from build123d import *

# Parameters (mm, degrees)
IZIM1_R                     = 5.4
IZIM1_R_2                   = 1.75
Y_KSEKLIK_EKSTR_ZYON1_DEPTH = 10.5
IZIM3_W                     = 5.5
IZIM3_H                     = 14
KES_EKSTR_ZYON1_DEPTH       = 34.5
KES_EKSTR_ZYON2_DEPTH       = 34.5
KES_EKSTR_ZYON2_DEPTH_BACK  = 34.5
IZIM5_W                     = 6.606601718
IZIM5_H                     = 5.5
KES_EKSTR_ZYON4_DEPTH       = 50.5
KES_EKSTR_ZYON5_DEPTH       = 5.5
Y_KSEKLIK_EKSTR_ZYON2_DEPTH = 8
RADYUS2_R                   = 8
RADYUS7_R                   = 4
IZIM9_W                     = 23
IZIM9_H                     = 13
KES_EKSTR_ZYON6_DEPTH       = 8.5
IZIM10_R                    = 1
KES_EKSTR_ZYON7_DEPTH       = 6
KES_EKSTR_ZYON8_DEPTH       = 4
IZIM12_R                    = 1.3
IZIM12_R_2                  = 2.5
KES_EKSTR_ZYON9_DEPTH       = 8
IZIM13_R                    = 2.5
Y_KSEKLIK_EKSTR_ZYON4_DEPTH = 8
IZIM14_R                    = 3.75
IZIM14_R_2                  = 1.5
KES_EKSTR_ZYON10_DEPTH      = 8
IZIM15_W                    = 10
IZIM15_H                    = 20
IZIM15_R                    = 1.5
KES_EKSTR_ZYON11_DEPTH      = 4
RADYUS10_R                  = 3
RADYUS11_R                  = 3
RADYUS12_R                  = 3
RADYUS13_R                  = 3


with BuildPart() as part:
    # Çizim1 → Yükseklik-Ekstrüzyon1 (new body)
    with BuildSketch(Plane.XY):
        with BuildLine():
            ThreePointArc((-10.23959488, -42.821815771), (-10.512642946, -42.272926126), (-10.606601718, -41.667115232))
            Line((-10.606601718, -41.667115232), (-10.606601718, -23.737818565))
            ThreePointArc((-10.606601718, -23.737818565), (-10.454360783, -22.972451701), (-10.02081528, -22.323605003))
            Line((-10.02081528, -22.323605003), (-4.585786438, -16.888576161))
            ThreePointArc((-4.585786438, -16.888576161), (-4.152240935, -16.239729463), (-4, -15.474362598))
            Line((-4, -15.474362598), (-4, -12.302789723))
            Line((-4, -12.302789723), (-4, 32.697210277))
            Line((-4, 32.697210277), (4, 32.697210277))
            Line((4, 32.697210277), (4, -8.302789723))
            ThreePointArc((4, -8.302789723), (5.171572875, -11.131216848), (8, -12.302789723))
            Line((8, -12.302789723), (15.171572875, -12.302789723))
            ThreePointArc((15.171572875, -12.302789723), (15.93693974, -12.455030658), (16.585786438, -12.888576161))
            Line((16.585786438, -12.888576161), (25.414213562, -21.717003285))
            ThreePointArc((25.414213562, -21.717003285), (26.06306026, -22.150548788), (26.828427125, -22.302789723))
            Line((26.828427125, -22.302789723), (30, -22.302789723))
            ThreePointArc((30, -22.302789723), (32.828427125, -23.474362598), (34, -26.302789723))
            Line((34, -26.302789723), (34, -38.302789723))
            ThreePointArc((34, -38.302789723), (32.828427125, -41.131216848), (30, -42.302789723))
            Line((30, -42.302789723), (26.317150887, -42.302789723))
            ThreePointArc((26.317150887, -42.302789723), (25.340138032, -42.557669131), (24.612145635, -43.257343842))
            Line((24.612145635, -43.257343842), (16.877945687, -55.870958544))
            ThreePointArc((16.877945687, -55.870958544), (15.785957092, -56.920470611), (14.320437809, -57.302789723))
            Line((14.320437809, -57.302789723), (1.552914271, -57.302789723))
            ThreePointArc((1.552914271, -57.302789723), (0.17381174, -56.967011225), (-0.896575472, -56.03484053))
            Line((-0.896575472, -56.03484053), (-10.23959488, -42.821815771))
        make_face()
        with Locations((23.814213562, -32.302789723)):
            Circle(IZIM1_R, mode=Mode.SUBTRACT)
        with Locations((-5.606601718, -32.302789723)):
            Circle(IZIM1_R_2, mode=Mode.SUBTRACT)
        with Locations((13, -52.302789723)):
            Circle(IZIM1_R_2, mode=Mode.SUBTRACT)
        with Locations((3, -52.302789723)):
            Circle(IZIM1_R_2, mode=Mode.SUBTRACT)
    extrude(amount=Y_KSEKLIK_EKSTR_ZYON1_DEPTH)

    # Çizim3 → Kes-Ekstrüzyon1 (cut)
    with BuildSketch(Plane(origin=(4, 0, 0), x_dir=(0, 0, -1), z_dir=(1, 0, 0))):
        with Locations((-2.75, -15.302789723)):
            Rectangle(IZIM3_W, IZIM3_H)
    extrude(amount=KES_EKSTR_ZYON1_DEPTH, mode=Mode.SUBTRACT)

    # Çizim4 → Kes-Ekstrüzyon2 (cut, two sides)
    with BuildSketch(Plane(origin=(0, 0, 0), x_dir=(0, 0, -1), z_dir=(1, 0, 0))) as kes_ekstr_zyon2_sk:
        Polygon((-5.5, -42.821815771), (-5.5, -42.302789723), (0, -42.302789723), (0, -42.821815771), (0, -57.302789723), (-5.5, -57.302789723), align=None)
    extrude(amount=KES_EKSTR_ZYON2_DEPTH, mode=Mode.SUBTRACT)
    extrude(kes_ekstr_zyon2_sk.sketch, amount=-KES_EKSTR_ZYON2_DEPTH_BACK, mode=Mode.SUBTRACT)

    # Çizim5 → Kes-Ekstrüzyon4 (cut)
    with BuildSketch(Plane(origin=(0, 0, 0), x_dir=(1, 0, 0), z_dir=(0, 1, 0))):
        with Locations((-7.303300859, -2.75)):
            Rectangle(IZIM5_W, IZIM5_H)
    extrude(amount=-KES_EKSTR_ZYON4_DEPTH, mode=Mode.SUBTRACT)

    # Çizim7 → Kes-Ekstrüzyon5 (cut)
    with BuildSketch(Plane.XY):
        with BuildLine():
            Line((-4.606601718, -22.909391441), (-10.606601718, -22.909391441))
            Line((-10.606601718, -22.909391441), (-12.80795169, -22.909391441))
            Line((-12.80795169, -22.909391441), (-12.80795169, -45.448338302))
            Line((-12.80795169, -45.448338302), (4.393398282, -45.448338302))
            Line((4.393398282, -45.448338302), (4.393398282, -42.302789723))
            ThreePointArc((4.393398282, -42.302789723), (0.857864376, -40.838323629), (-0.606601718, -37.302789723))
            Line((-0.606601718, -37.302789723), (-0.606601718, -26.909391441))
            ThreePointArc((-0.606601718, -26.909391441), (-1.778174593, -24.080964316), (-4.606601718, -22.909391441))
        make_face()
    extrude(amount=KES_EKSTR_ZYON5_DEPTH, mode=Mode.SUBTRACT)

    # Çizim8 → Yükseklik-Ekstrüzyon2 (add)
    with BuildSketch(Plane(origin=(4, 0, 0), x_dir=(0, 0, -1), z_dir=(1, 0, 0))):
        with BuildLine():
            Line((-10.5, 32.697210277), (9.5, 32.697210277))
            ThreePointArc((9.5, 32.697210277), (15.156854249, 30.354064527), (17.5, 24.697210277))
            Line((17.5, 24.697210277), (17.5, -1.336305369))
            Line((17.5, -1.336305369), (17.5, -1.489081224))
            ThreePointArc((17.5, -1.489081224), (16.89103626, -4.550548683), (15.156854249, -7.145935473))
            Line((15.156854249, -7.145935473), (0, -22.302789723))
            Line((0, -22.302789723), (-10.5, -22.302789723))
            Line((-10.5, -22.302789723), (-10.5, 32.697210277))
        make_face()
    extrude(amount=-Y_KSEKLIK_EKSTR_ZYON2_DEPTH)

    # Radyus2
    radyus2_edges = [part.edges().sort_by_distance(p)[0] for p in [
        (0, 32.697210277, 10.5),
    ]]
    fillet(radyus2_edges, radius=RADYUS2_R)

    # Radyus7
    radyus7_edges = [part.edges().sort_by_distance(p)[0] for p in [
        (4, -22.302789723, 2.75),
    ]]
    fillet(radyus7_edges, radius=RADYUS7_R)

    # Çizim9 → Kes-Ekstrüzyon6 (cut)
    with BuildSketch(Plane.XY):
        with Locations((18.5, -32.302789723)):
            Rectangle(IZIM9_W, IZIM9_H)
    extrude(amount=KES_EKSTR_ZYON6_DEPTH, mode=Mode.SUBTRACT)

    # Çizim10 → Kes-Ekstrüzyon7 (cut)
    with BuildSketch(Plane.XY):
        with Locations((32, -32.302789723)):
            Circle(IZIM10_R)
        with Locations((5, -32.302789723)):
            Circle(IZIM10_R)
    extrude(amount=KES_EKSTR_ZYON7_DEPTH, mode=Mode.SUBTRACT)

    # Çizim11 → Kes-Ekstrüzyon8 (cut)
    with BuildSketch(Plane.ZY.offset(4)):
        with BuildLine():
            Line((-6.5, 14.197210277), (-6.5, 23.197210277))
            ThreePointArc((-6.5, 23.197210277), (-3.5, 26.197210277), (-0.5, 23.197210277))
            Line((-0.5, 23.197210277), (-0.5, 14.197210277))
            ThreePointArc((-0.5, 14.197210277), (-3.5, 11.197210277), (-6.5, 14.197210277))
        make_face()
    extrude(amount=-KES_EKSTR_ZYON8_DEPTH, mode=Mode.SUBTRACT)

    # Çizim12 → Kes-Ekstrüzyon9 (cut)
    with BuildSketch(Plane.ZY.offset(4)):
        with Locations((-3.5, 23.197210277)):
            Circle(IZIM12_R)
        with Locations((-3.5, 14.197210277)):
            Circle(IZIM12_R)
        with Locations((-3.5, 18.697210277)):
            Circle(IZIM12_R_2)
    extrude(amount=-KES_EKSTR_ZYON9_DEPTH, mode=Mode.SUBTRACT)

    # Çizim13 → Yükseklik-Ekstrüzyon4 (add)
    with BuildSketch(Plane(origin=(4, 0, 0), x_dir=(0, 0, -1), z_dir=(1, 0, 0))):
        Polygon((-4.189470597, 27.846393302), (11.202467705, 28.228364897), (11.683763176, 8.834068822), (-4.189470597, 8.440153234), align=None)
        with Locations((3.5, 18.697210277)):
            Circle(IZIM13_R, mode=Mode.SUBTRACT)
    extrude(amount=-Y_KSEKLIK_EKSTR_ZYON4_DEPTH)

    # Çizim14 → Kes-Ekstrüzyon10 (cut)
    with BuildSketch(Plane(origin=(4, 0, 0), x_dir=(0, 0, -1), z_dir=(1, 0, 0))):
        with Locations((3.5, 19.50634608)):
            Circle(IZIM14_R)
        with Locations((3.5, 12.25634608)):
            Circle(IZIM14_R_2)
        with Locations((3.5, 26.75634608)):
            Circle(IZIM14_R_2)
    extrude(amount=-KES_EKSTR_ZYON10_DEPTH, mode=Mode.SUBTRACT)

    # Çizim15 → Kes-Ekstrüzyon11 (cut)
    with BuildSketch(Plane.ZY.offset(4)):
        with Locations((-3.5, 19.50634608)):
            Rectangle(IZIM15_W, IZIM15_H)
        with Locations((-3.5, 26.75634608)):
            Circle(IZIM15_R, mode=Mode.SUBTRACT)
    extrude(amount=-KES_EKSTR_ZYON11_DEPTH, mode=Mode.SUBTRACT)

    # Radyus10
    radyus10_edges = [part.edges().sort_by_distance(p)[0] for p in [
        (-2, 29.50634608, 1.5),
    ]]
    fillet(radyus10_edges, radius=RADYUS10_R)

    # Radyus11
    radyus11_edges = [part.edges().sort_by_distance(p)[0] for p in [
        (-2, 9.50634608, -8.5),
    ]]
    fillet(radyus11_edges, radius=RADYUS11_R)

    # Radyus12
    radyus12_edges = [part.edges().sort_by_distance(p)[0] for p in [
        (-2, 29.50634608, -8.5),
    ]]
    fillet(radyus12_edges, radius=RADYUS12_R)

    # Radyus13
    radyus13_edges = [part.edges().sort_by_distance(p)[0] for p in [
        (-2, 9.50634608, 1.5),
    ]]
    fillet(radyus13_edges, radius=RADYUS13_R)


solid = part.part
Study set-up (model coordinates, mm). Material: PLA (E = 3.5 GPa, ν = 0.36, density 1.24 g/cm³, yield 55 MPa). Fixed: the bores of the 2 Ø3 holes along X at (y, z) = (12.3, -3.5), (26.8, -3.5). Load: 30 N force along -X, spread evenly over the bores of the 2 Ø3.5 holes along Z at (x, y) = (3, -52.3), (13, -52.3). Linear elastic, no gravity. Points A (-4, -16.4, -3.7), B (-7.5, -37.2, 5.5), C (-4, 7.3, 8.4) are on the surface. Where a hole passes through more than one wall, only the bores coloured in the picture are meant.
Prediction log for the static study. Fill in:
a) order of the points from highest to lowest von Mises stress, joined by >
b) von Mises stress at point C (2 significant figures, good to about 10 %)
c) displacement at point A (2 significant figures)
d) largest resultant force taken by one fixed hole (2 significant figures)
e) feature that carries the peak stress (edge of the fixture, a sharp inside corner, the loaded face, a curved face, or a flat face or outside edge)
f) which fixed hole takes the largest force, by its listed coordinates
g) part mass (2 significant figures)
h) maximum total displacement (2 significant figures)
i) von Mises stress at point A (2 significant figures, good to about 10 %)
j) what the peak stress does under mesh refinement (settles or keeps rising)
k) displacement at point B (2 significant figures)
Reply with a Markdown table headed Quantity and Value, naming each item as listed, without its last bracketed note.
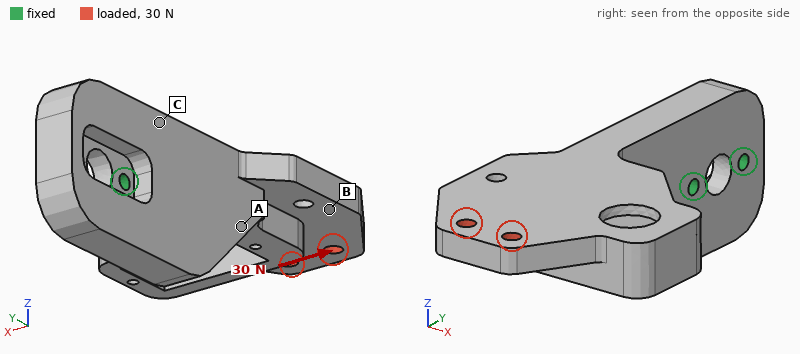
| Quantity | Value |
|---|---|
| order of the points from highest to lowest von Mises stress, joined by > | C > A > B |
| von Mises stress at point C | 7.3 MPa |
| displacement at point A | 0.31 mm |
| largest resultant force taken by one fixed hole | 130 N |
| feature that carries the peak stress | edge of the fixture |
| which fixed hole takes the largest force, by its listed coordinates | (12.3, -3.5) |
| part mass | 22 g |
| maximum total displacement | 1.2 mm |
| von Mises stress at point A | 4.7 MPa |
| what the peak stress does under mesh refinement | keeps rising |
| displacement at point B | 0.75 mm |
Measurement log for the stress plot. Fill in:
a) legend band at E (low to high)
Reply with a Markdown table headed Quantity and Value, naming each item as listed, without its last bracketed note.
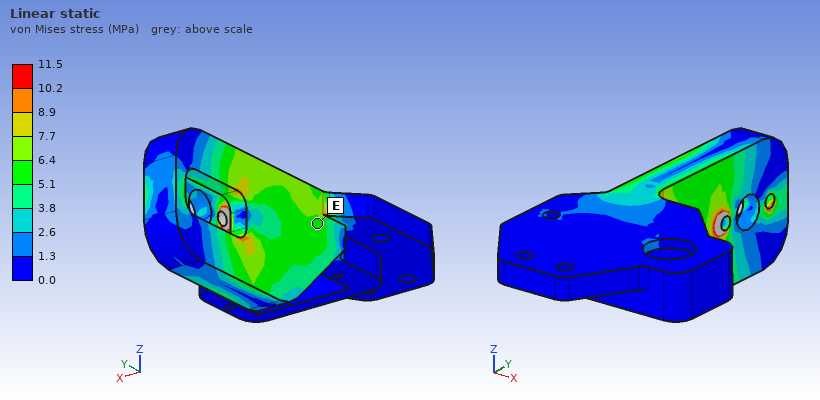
| Quantity | Value |
|---|---|
| legend band at E | 5.1 to 6.4 MPa |
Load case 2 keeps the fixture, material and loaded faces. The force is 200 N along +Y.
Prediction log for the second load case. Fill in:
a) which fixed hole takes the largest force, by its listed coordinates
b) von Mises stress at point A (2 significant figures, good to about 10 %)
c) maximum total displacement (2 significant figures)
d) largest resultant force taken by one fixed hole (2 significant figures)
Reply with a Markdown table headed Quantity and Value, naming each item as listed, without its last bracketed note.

| Quantity | Value |
|---|---|
| which fixed hole takes the largest force, by its listed coordinates | (12.3, -3.5) |
| von Mises stress at point A | 6.0 MPa |
| maximum total displacement | 1.1 mm |
| largest resultant force taken by one fixed hole | 230 N |
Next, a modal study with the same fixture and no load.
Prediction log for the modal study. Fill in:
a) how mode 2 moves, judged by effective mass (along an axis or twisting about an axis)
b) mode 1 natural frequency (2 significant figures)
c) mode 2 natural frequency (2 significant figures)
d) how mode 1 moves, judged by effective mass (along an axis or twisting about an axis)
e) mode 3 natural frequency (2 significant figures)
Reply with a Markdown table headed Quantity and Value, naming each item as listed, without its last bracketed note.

| Quantity | Value |
|---|---|
| how mode 2 moves, judged by effective mass | along Z |
| mode 1 natural frequency | 350 Hz |
| mode 2 natural frequency | 640 Hz |
| how mode 1 moves, judged by effective mass | along X |
| mode 3 natural frequency | 1100 Hz |
